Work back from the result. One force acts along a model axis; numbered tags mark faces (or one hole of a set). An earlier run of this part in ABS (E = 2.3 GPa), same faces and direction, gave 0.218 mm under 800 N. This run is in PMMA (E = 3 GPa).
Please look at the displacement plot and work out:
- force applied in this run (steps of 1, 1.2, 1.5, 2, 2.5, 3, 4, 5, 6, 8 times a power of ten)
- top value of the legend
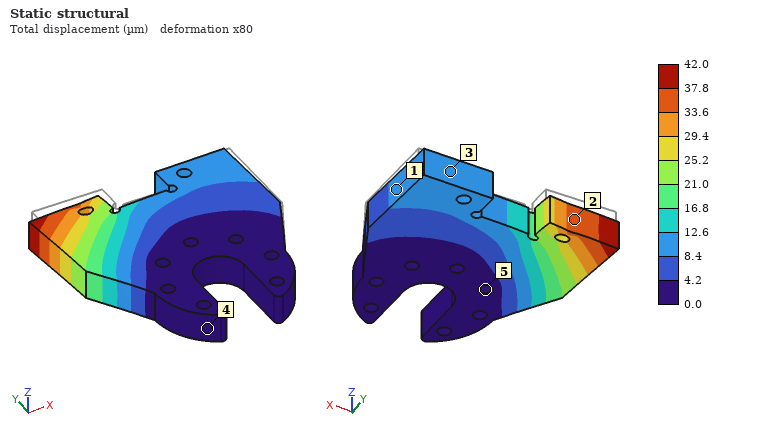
200 N
42.0 µm
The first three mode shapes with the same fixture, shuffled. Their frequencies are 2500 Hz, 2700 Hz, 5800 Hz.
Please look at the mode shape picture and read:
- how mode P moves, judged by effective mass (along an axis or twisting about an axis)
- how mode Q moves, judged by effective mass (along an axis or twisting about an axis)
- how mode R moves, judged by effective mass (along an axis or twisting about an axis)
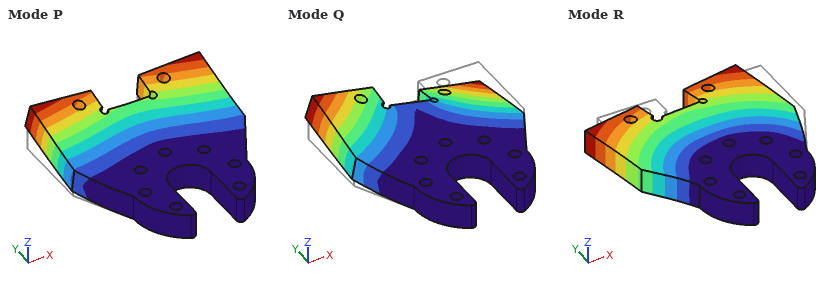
along Z
twisting about Y
along X
